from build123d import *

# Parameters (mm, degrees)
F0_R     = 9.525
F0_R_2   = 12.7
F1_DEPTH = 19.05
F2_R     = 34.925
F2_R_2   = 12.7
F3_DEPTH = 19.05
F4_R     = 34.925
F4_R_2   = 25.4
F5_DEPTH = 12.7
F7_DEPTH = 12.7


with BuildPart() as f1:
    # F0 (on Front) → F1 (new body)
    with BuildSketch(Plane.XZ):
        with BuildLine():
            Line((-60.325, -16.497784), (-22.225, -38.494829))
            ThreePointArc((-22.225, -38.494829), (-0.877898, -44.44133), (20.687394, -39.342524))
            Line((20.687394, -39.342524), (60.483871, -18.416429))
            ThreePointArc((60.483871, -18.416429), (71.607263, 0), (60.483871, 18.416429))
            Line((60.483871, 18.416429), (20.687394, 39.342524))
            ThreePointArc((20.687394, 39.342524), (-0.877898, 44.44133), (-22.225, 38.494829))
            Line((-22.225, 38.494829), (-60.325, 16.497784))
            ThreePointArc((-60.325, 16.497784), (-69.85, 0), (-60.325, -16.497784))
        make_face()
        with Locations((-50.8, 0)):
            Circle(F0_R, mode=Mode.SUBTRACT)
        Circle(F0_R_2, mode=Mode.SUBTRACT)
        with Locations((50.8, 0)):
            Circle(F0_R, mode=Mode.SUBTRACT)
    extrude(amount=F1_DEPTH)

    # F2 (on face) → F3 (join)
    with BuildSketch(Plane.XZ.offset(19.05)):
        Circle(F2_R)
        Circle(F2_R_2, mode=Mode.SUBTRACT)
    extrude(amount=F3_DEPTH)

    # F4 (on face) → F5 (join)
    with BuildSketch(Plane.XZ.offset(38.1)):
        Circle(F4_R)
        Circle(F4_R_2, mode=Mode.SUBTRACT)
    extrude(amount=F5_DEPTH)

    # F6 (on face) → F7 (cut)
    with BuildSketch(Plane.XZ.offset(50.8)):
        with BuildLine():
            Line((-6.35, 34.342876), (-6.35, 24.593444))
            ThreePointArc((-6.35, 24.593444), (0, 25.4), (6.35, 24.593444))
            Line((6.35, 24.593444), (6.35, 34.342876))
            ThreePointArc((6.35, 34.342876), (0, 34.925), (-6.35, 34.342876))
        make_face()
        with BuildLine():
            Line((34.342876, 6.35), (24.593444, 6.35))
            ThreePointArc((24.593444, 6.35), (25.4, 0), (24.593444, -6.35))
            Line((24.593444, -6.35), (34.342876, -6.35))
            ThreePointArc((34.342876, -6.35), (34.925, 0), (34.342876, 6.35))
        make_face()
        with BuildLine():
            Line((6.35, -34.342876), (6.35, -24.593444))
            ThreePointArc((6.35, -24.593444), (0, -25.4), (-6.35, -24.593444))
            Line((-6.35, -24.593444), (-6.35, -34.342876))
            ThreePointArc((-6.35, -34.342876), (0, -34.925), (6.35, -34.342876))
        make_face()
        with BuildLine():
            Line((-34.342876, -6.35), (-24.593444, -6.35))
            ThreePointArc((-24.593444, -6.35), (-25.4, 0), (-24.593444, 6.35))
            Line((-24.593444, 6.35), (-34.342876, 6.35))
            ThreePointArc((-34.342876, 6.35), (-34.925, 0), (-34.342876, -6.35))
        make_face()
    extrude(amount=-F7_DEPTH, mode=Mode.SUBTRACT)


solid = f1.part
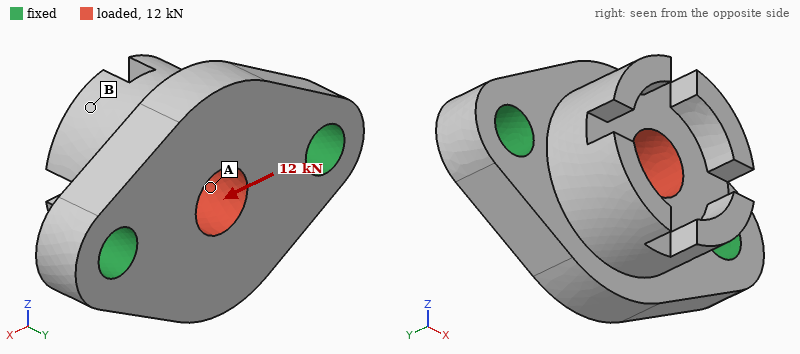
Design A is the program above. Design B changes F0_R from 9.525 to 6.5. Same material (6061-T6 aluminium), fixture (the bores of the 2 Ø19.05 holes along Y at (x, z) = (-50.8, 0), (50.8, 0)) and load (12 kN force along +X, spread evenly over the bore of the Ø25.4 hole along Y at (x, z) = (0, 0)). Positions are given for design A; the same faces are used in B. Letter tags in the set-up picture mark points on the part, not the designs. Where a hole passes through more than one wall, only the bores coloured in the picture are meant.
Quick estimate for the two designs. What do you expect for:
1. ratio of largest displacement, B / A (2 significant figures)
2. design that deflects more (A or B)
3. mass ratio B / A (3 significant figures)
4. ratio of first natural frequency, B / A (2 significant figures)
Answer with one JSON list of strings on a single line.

["1.2", "B", "1.03", "0.86"]
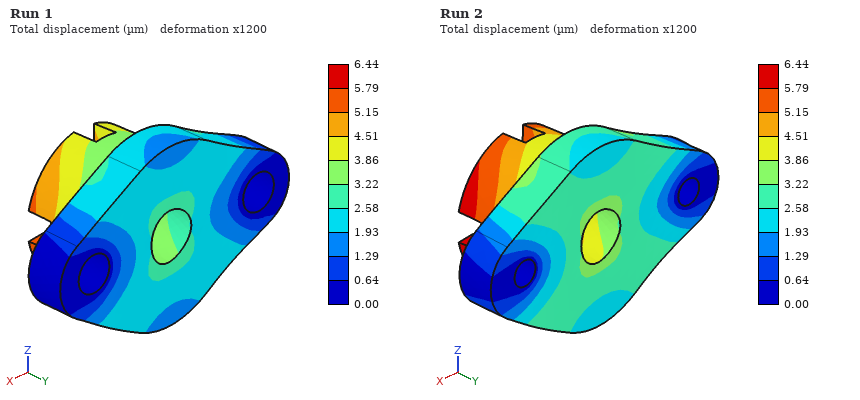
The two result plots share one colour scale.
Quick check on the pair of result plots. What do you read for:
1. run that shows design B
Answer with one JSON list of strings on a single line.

["Run 2"]
